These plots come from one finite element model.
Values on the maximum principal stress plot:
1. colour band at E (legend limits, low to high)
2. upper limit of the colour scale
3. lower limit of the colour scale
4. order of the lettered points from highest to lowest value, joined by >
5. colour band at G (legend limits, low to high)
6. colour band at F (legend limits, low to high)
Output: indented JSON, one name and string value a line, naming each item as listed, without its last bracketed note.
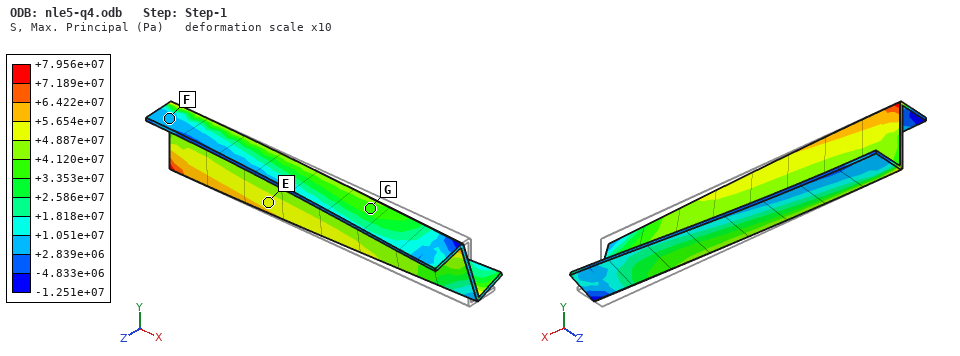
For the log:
{
  "colour band at E": "+4.887e+07 to +5.654e+07 Pa",
  "upper limit of the colour scale": "+7.956e+07 Pa",
  "lower limit of the colour scale": "-1.251e+07 Pa",
  "order of the lettered points from highest to lowest value, joined by >": "E > G > F",
  "colour band at G": "+3.353e+07 to +4.120e+07 Pa",
  "colour band at F": "+2.839e+06 to +1.051e+07 Pa"
}
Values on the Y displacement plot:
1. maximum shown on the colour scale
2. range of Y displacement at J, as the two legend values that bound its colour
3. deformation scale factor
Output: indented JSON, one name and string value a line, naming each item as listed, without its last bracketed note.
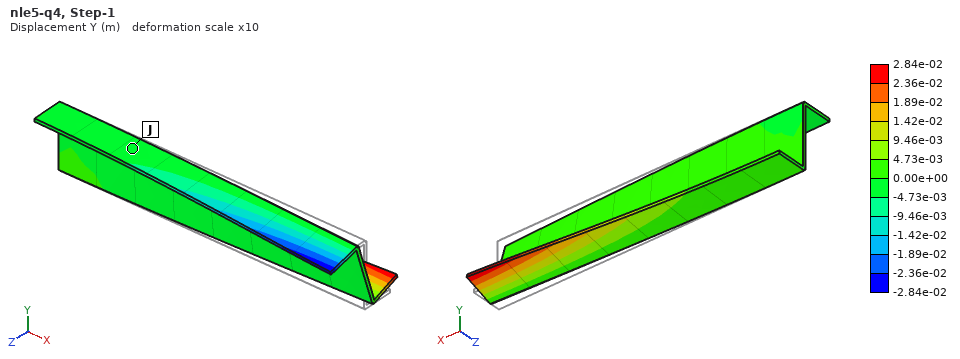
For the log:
{
  "maximum shown on the colour scale": "2.84e-02 m",
  "range of Y displacement at J, as the two legend values that bound its colour": "-4.73e-03 to 0.00e+00 m",
  "deformation scale factor": "10"
}
